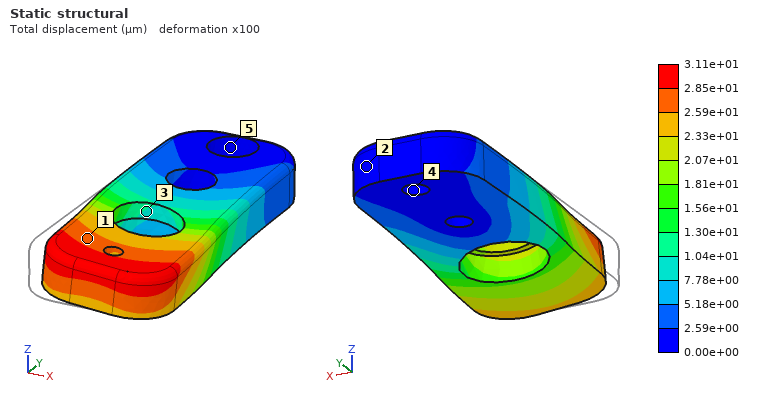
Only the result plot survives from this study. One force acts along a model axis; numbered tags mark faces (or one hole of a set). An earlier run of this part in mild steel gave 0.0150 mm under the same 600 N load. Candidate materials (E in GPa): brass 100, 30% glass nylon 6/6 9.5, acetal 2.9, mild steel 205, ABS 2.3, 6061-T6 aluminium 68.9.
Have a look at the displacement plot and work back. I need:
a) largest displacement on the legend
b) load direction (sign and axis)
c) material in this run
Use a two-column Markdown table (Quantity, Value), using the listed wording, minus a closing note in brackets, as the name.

| Quantity | Value |
|---|---|
| largest displacement on the legend | 3.11e+01 µm |
| load direction | +X |
| material in this run | brass |
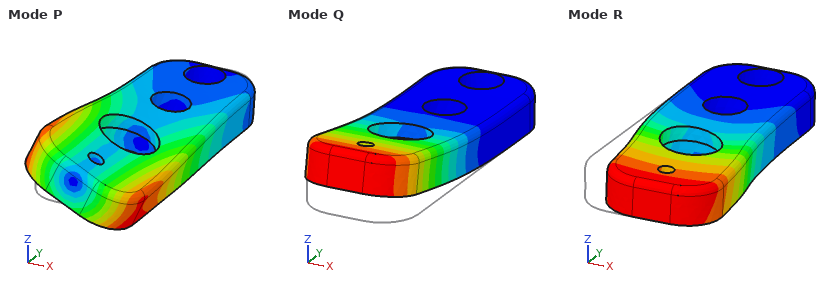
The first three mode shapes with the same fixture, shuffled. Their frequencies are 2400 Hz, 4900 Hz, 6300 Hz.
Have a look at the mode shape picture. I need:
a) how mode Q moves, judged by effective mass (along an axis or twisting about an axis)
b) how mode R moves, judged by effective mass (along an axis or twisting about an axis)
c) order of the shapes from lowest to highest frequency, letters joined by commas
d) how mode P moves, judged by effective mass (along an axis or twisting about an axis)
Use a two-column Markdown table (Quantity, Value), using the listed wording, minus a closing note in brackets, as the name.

| Quantity | Value |
|---|---|
| how mode Q moves, judged by effective mass | along Z |
| how mode R moves, judged by effective mass | along X |
| order of the shapes from lowest to highest frequency, letters joined by commas | Q, R, P |
| how mode P moves, judged by effective mass | twisting about Y |
